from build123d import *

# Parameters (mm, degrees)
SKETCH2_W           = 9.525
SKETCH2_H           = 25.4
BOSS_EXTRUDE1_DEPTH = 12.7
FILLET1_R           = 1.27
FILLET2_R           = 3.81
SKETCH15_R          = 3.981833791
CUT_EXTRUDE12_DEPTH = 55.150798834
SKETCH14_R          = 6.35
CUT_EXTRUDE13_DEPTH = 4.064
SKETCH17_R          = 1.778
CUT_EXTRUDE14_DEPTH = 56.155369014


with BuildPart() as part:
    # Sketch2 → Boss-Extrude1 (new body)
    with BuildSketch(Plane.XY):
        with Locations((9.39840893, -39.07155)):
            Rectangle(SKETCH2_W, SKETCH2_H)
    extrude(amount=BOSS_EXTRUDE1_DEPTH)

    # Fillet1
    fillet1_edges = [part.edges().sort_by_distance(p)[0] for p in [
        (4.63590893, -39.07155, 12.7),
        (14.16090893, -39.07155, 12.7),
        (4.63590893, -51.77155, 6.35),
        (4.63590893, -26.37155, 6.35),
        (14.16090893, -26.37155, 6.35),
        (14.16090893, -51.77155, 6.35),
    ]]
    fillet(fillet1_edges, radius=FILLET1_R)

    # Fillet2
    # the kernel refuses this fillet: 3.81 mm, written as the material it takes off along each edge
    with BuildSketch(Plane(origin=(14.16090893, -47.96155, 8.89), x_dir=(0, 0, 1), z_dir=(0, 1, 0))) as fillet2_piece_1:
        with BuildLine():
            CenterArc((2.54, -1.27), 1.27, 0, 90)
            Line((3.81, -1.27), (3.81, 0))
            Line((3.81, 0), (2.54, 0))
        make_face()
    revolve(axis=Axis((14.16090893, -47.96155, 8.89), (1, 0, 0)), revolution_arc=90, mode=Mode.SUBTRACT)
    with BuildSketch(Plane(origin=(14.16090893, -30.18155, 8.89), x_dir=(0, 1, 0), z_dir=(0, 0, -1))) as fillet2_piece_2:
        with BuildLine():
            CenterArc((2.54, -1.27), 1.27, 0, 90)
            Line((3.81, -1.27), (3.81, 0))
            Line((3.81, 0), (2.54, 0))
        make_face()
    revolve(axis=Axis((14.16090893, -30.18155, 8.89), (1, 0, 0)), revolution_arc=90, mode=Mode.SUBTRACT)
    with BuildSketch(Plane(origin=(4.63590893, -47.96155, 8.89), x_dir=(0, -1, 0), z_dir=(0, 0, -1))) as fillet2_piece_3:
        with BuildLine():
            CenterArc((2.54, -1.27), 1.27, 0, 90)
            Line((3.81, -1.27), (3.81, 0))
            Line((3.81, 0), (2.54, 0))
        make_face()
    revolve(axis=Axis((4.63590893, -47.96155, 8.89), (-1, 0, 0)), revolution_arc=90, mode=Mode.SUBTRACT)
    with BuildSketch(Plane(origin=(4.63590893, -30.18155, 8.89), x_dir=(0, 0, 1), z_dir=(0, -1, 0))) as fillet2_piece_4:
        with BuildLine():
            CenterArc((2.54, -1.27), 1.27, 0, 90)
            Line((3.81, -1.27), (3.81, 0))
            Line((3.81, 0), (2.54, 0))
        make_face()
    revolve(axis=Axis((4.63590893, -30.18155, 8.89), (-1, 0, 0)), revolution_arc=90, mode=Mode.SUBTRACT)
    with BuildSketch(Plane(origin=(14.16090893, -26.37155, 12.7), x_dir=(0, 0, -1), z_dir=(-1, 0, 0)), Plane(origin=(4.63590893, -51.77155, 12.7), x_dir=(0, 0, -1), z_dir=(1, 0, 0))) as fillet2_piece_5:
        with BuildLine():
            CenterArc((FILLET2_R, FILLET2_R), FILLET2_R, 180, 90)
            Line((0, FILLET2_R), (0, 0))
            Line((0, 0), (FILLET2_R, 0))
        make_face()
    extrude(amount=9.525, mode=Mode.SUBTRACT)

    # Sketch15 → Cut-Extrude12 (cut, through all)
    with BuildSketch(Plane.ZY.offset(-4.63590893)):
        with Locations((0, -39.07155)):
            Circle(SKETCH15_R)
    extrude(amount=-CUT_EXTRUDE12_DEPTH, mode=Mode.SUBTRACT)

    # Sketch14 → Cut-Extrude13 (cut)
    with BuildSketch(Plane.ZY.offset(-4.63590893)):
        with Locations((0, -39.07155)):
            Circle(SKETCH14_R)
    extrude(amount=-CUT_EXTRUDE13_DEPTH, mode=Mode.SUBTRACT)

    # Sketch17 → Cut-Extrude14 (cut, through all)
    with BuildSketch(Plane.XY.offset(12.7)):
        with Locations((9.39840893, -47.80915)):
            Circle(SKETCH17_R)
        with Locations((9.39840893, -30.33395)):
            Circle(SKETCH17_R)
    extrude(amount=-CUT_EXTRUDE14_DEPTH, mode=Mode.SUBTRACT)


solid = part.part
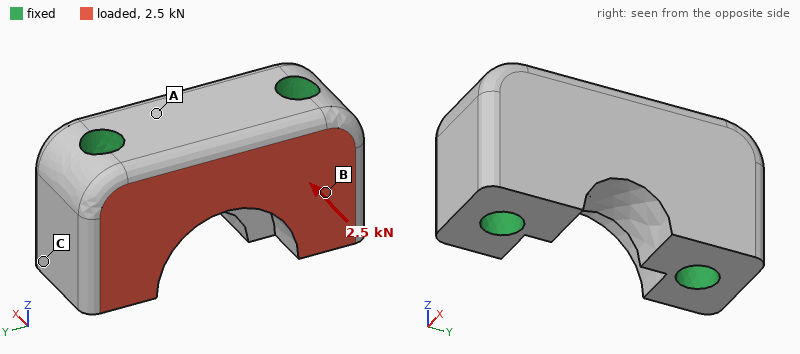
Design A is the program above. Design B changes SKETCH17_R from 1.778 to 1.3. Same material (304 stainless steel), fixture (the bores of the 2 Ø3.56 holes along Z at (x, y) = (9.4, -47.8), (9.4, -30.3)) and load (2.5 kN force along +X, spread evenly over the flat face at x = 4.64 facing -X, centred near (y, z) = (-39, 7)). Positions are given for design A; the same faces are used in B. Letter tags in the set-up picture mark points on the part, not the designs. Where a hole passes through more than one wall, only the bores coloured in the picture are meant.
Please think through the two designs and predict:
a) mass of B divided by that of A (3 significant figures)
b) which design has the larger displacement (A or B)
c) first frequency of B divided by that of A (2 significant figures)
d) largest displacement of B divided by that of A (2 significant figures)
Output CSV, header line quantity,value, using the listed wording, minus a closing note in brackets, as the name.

quantity,value
mass of B divided by that of A,1.05
which design has the larger displacement,B
first frequency of B divided by that of A,0.86
largest displacement of B divided by that of A,1.2
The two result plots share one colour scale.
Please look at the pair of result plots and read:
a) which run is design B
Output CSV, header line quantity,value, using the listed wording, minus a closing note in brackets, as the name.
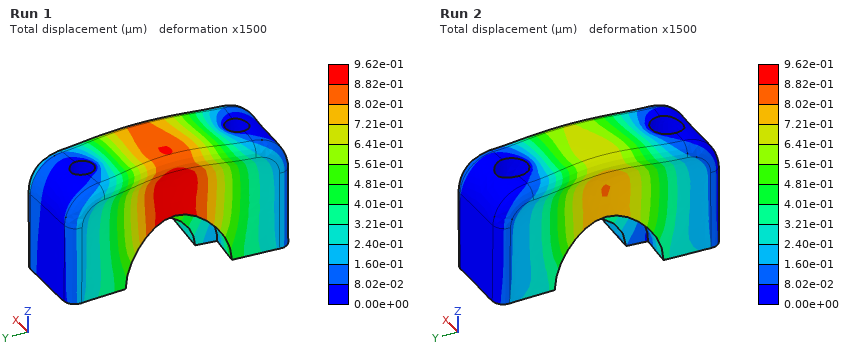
quantity,value
which run is design B,Run 1
